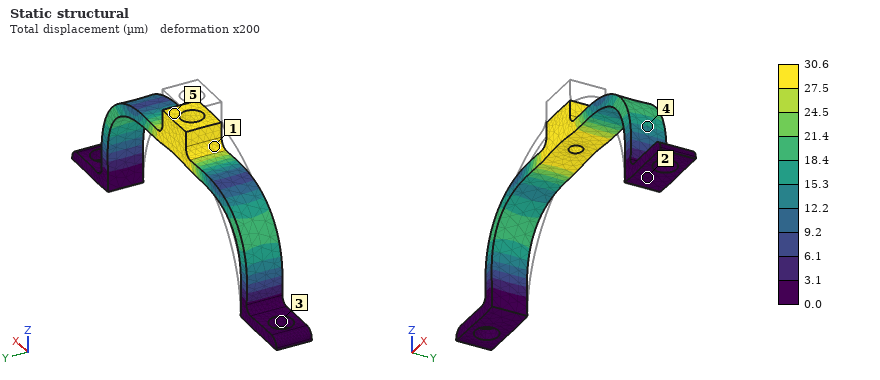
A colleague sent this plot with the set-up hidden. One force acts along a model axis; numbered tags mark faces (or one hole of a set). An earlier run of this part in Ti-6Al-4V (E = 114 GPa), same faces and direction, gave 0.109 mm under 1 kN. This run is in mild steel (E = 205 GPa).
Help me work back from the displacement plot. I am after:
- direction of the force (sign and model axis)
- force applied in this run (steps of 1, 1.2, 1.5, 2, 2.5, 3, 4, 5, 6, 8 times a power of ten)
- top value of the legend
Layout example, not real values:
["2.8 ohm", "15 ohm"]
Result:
["-Z", "500 N", "30.6 µm"]
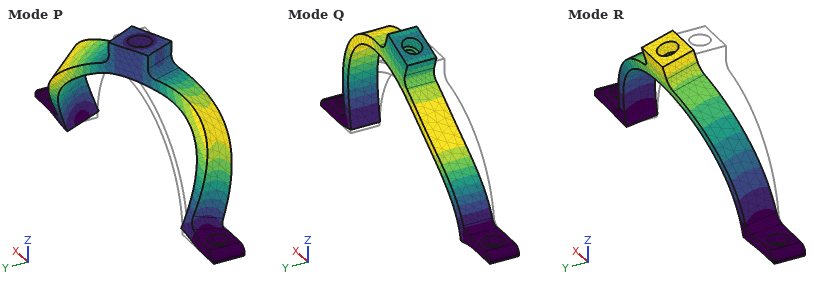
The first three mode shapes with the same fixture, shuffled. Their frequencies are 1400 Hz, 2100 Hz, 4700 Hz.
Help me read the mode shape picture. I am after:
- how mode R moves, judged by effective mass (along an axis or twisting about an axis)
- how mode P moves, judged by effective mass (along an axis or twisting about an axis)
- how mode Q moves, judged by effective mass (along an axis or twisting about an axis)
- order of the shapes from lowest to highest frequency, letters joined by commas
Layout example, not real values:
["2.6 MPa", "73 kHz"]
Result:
["along Y", "twisting about Z", "along X", "R, Q, P"]
